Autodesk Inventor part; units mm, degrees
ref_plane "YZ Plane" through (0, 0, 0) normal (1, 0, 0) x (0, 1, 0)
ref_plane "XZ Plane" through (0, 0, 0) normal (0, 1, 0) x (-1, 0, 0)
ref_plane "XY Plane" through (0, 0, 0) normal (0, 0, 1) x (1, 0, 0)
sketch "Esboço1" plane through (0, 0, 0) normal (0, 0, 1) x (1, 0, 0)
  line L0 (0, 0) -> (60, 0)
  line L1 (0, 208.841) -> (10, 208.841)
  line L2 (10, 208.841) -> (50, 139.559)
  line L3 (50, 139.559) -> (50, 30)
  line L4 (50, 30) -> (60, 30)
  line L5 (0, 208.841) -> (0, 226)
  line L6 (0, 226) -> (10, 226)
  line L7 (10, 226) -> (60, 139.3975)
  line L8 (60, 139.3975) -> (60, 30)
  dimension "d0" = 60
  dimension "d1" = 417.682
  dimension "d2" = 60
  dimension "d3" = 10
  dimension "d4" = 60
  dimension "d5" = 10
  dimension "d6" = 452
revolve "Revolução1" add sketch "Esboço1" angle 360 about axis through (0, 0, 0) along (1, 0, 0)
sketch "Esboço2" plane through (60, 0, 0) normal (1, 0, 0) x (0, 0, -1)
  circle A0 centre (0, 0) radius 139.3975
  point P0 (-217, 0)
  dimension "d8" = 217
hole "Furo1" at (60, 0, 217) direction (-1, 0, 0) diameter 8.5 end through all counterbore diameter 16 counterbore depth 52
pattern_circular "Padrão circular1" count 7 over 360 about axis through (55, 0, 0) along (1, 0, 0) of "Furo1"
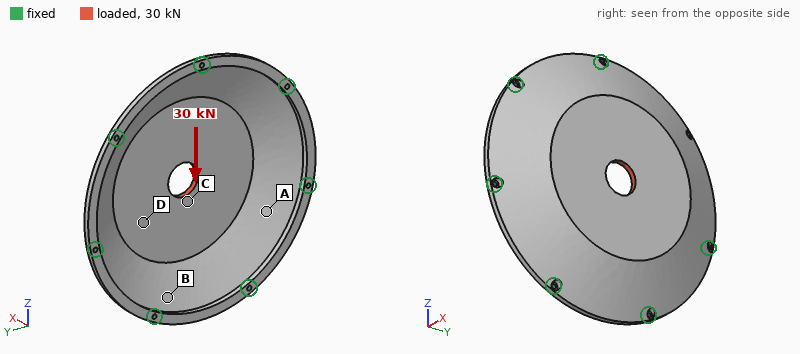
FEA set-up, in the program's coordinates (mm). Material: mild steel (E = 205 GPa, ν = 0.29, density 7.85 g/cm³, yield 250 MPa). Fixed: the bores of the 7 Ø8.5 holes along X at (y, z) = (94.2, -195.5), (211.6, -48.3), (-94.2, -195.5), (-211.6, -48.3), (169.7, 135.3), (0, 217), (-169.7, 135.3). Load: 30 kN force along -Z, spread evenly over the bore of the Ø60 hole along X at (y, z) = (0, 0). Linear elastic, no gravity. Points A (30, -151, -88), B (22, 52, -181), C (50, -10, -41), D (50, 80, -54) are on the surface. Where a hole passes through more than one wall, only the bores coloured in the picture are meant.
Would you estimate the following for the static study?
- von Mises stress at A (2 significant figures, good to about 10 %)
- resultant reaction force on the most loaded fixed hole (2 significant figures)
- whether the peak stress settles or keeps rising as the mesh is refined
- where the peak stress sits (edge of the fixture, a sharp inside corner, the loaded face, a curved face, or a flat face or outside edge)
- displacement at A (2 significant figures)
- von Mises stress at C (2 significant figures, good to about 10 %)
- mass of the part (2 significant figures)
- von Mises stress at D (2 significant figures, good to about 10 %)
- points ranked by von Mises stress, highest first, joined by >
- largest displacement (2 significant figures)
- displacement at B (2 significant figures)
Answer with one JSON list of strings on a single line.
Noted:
["8.7 MPa", "5.4 kN", "keeps rising", "edge of the fixture", "6.5 µm", "17 MPa", "13 kg", "12 MPa", "C > D > A > B", "27 µm", "6.5 µm"]
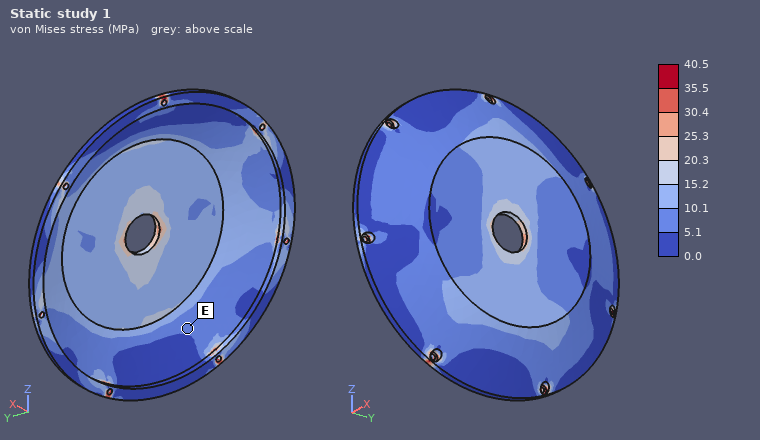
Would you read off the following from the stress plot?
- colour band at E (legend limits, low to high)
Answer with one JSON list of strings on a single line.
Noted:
["5.1 to 10.1 MPa"]
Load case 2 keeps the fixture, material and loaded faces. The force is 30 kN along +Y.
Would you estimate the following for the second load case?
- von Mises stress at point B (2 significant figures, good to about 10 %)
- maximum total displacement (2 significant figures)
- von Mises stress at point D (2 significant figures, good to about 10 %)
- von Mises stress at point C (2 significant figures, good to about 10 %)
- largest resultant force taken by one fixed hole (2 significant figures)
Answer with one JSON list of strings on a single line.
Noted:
["11 MPa", "27 µm", "13 MPa", "17 MPa", "5.5 kN"]
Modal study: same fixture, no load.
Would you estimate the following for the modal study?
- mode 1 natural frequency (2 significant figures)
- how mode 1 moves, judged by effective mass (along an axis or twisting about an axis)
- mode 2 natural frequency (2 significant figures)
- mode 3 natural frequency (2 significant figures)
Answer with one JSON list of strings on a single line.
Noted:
["880 Hz", "along X", "1600 Hz", "1600 Hz"]
